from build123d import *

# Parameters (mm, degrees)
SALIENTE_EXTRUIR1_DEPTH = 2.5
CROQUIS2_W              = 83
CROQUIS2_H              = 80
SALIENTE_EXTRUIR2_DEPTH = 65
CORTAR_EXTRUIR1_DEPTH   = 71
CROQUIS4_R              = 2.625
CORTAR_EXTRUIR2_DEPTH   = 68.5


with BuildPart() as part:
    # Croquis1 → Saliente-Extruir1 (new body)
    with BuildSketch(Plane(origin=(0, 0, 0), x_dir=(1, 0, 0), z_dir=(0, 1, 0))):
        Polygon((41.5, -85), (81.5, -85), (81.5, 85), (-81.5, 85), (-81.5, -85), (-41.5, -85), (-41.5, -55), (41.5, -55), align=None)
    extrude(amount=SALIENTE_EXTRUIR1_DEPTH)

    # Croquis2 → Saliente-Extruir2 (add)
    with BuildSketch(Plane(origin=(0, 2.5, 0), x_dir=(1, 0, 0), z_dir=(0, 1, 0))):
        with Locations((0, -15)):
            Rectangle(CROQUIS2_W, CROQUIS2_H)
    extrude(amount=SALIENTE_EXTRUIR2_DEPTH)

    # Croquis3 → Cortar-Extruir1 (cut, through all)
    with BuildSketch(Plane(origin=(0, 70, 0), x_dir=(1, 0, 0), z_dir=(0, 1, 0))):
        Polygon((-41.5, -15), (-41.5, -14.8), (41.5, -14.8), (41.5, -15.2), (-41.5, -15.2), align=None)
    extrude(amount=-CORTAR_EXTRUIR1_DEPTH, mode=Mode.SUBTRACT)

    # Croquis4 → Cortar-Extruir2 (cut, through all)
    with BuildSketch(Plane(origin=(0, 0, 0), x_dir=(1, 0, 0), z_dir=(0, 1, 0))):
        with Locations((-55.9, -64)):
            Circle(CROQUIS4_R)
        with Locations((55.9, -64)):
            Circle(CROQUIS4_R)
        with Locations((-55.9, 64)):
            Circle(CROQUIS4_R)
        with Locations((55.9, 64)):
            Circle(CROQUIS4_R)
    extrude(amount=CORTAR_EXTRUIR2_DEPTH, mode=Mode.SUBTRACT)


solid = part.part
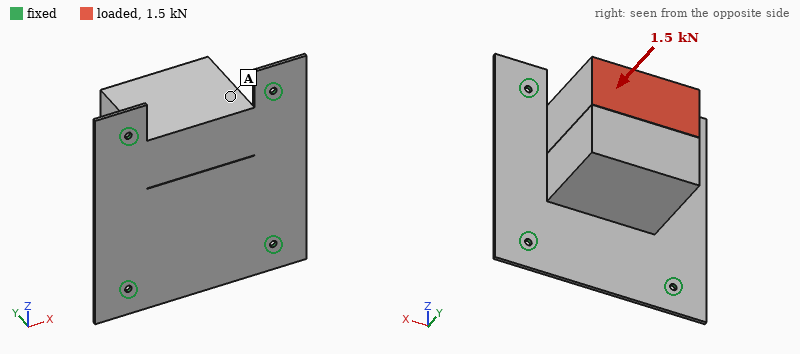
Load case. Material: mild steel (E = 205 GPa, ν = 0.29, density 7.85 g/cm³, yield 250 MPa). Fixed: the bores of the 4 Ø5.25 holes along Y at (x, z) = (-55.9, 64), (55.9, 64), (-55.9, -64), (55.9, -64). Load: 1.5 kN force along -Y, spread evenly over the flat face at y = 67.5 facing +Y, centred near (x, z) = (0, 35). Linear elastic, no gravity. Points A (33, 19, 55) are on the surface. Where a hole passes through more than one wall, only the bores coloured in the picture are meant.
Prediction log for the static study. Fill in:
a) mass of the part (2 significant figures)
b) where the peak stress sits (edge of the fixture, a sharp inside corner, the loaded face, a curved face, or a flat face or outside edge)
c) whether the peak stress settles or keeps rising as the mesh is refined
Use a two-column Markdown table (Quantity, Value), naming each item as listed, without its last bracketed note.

| Quantity | Value |
|---|---|
| mass of the part | 3.9 kg |
| where the peak stress sits | a sharp inside corner |
| whether the peak stress settles or keeps rising as the mesh is refined | keeps rising |
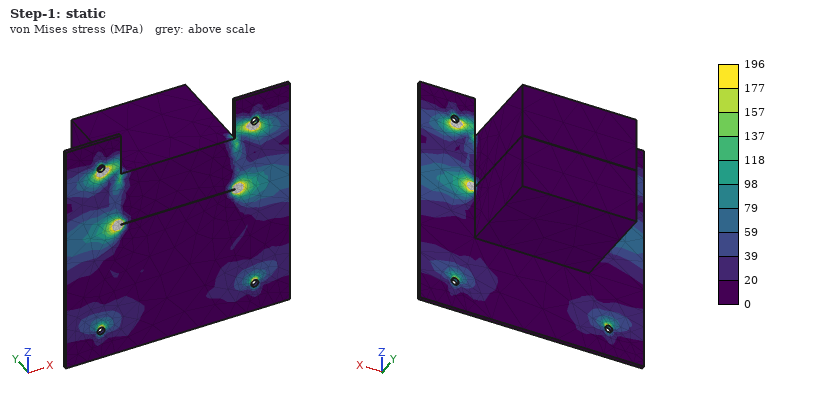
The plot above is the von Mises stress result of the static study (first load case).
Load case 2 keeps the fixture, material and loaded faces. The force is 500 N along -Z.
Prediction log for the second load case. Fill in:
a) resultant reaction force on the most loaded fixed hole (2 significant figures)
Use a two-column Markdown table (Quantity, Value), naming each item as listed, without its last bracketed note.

| Quantity | Value |
|---|---|
| resultant reaction force on the most loaded fixed hole | 250 N |
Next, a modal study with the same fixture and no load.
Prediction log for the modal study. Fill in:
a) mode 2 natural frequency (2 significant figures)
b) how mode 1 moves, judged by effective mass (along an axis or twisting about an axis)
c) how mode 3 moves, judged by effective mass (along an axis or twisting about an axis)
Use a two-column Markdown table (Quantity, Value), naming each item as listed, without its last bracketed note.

| Quantity | Value |
|---|---|
| mode 2 natural frequency | 330 Hz |
| how mode 1 moves, judged by effective mass | along Y |
| how mode 3 moves, judged by effective mass | along X |
